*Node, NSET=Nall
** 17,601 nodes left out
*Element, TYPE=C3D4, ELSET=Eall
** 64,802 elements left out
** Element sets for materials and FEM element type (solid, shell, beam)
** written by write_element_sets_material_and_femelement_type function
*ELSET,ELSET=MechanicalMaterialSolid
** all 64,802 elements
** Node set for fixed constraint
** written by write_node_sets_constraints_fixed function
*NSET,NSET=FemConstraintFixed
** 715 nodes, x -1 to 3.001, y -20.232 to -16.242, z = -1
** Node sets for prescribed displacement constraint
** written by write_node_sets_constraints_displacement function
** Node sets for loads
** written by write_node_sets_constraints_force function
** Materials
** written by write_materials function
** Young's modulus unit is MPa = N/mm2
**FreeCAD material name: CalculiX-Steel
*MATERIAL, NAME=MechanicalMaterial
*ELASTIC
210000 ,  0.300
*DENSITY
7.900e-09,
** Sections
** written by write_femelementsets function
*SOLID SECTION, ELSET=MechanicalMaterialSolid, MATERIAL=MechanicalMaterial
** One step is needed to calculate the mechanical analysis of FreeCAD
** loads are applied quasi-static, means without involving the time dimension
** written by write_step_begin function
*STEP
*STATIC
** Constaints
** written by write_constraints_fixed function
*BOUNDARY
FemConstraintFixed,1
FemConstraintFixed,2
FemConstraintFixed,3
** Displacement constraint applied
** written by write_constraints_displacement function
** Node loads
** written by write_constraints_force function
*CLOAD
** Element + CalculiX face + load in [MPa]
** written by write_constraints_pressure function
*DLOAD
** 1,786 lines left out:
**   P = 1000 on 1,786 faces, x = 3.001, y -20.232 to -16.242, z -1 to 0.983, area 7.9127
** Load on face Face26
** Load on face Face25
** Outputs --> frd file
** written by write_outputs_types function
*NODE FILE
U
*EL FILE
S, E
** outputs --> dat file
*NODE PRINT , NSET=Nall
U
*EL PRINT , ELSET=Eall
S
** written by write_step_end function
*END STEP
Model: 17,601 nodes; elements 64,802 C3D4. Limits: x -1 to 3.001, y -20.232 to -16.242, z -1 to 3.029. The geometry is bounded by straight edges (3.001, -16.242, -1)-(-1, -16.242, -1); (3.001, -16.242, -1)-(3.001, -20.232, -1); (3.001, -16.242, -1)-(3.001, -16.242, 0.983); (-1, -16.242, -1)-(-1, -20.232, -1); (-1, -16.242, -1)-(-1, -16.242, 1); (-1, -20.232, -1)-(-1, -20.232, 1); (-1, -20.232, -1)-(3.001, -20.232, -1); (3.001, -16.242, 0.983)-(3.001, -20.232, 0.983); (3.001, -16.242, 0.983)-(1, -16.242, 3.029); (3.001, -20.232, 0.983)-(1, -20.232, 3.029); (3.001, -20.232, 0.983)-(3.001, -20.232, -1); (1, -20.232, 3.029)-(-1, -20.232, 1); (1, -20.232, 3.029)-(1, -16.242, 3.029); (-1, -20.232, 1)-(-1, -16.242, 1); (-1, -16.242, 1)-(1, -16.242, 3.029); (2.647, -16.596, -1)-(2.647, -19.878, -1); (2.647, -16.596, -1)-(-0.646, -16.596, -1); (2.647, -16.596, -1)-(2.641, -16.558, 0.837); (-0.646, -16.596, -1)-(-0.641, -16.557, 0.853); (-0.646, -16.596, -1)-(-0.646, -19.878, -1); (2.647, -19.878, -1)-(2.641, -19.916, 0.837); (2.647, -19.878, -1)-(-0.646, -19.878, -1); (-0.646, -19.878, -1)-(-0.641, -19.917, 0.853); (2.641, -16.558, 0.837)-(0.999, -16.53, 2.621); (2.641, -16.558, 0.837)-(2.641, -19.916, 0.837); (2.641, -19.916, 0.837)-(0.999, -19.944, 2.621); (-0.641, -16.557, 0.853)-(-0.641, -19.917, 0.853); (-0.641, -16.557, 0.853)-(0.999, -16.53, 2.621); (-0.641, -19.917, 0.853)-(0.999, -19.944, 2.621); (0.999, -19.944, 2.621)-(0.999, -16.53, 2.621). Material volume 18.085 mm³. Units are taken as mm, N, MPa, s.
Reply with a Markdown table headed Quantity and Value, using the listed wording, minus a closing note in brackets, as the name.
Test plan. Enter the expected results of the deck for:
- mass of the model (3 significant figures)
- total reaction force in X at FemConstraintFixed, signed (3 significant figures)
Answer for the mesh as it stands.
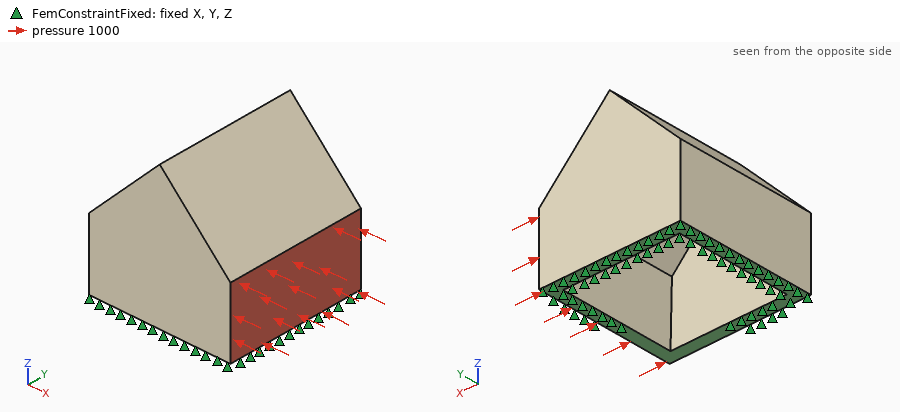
| Quantity | Value |
|---|---|
| mass of the model | 1.43e-04 kg |
| total reaction force in X at FemConstraintFixed, signed | 7910 N |
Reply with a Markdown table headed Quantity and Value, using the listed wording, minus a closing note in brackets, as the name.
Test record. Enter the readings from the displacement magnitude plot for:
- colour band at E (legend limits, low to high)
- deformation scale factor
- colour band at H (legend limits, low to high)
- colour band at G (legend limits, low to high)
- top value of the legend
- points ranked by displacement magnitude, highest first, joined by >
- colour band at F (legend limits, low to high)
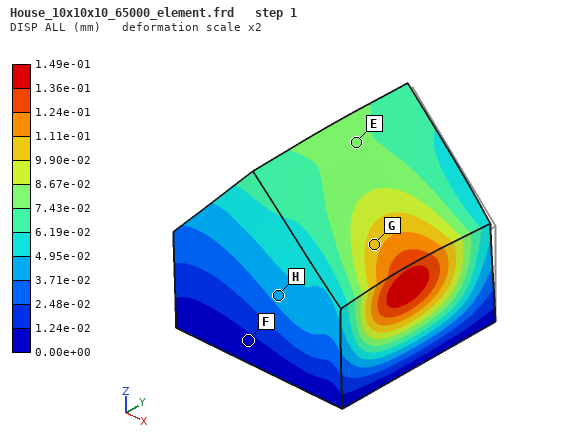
| Quantity | Value |
|---|---|
| colour band at E | 7.43e-02 to 8.67e-02 mm |
| deformation scale factor | 2 |
| colour band at H | 3.71e-02 to 4.95e-02 mm |
| colour band at G | 9.90e-02 to 1.11e-01 mm |
| top value of the legend | 1.49e-01 mm |
| points ranked by displacement magnitude, highest first, joined by > | G > E > H > F |
| colour band at F | 0.00e+00 to 1.24e-02 mm |
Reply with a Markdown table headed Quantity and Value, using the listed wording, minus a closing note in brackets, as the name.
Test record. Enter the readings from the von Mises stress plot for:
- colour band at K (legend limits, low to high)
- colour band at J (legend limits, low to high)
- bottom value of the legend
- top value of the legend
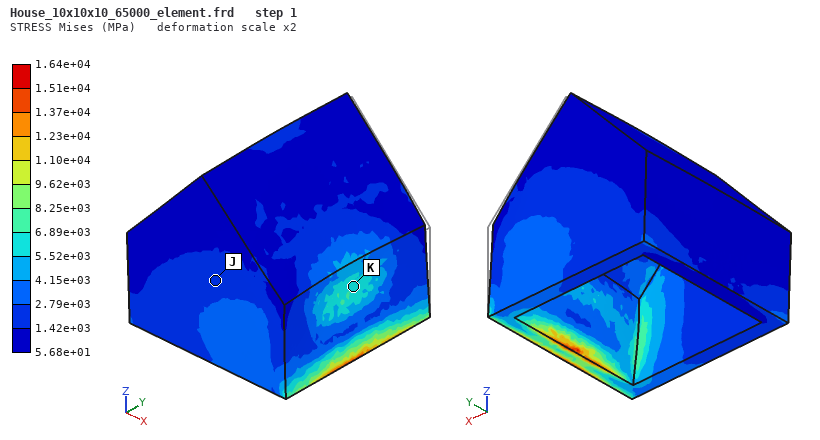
| Quantity | Value |
|---|---|
| colour band at K | 5.52e+03 to 6.89e+03 MPa |
| colour band at J | 1.42e+03 to 2.79e+03 MPa |
| bottom value of the legend | 5.68e+01 MPa |
| top value of the legend | 1.64e+04 MPa |
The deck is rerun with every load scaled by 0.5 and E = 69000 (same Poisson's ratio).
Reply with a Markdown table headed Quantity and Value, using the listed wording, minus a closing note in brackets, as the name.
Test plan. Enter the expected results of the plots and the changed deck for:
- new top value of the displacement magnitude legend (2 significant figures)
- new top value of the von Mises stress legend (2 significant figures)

| Quantity | Value |
|---|---|
| new top value of the displacement magnitude legend | 0.23 mm |
| new top value of the von Mises stress legend | 8200 MPa |
